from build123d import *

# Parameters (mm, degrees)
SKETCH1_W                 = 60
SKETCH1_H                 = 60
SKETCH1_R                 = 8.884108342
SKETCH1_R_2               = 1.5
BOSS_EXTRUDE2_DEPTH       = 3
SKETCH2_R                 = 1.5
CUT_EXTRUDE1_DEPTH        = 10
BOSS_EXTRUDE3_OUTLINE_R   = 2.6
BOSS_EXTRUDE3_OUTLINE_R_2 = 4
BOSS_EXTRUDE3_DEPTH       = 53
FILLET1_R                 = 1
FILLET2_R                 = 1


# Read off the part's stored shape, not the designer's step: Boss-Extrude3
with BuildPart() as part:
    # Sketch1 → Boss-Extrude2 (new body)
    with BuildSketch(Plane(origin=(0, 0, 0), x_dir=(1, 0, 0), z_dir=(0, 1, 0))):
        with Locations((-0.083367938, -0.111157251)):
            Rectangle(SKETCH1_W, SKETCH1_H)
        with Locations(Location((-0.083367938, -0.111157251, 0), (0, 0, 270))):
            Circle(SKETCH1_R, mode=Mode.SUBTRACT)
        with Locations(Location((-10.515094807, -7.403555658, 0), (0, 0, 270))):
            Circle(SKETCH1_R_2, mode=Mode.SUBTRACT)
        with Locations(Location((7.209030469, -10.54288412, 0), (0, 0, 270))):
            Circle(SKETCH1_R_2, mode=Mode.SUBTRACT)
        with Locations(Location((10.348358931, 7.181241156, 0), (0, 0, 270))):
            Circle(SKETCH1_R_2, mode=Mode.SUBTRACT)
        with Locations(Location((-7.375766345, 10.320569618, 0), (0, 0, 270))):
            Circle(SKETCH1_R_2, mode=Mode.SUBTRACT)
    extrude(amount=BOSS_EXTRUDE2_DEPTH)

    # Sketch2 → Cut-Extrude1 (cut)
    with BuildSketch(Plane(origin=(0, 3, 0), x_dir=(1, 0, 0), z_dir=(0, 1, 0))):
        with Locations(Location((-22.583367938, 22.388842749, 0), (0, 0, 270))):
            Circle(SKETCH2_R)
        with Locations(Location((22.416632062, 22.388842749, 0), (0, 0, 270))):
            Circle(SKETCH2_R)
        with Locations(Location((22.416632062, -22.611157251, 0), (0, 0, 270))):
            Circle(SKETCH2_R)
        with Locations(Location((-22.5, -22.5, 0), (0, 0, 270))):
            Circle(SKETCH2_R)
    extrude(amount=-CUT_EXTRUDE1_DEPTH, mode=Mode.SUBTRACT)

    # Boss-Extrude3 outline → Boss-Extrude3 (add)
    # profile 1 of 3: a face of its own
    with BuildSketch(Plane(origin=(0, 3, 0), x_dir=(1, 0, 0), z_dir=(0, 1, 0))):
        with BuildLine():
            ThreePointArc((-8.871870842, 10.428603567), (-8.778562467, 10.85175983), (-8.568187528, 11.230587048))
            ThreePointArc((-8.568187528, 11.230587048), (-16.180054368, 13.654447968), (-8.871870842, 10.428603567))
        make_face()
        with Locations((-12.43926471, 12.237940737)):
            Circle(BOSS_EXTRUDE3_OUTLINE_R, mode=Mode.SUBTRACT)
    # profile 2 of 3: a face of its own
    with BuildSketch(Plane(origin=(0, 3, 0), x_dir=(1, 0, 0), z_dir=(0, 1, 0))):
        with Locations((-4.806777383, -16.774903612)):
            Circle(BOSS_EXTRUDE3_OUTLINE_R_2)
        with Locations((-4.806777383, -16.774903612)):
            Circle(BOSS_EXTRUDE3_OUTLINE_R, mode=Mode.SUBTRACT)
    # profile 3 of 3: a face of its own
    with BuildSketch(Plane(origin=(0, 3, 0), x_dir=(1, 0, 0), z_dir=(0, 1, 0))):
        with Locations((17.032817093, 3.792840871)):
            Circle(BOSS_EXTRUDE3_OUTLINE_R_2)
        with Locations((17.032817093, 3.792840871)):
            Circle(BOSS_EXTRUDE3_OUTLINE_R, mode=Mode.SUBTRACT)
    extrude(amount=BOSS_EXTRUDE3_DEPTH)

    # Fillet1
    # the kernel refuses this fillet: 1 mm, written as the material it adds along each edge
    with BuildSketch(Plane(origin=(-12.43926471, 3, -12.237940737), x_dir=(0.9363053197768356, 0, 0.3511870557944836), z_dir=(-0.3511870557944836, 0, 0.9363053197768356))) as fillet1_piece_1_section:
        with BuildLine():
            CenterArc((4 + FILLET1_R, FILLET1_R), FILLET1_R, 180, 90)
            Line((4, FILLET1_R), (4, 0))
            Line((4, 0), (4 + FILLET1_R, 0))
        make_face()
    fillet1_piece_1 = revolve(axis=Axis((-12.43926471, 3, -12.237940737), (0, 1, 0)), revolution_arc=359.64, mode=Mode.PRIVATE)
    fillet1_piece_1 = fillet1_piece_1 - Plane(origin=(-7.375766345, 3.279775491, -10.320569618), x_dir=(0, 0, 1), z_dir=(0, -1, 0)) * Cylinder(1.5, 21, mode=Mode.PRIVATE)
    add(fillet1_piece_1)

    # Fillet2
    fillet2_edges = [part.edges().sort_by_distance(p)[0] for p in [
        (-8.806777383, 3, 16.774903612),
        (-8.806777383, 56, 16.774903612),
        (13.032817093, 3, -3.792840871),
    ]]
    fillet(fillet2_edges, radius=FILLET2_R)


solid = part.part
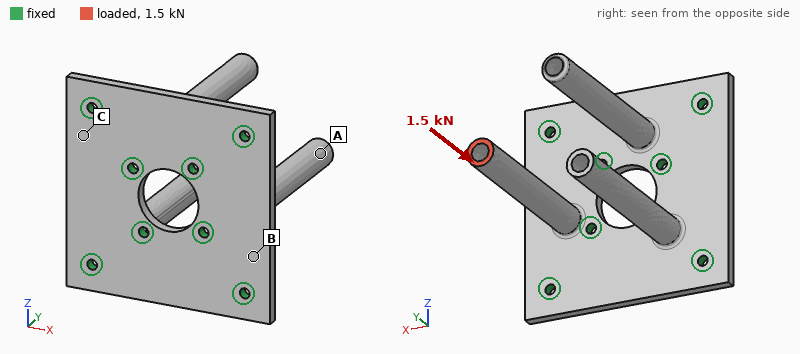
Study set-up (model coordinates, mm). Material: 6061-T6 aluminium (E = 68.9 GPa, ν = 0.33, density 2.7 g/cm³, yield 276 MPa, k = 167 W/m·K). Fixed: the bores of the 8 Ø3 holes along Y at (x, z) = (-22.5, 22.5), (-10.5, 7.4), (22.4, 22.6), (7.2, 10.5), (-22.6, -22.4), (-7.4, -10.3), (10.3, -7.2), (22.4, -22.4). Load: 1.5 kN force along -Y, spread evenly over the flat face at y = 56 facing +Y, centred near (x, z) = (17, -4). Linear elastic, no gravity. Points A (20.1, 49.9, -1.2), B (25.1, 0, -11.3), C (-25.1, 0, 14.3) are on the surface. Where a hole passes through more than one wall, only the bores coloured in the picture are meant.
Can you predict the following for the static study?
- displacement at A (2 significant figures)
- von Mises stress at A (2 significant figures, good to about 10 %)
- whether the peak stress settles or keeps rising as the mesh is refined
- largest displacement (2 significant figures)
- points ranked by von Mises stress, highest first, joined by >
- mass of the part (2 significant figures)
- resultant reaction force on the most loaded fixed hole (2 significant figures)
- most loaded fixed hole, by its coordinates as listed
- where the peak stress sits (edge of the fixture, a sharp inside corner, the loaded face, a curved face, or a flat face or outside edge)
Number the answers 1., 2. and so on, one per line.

1. 0.25 mm
2. 52 MPa
3. keeps rising
4. 0.28 mm
5. A > B > C
6. 39 g
7. 1.1 kN
8. (10.3, -7.2)
9. edge of the fixture
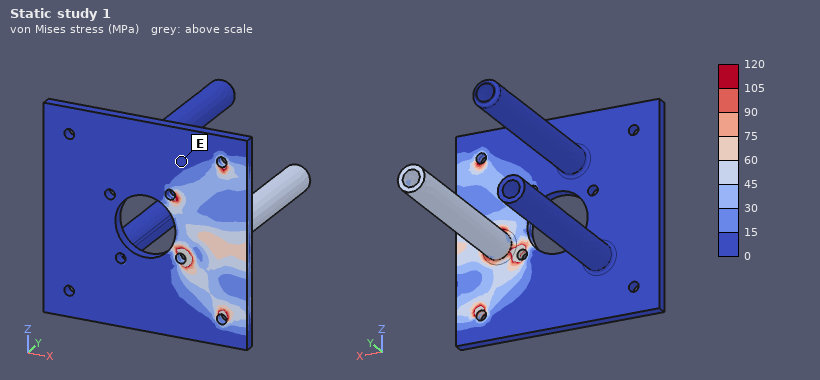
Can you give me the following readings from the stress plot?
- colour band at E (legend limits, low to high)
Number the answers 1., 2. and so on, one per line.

1. 0 to 15 MPa
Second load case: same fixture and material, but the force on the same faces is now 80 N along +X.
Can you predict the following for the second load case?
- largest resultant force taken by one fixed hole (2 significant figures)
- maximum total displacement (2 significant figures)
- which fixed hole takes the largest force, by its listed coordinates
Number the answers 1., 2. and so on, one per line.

1. 170 N
2. 0.55 mm
3. (10.3, -7.2)
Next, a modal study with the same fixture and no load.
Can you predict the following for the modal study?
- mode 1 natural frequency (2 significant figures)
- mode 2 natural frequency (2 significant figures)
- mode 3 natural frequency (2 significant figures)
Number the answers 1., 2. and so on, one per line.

1. 1800 Hz
2. 1800 Hz
3. 2000 Hz
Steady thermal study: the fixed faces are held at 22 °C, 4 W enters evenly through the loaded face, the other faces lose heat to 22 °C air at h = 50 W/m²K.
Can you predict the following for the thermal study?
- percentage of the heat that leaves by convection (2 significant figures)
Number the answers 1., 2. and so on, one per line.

1. 44 %
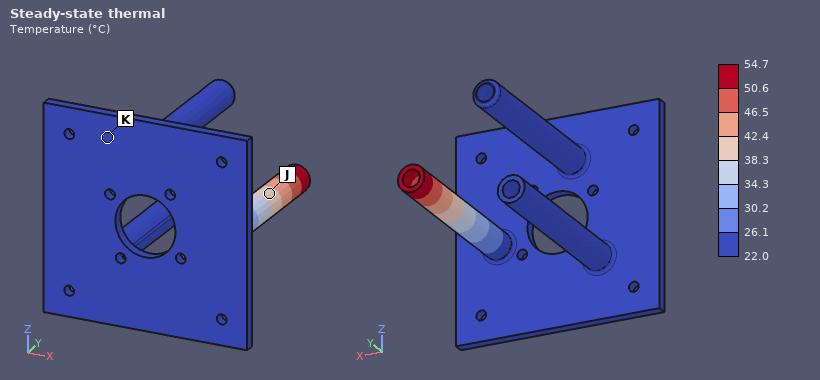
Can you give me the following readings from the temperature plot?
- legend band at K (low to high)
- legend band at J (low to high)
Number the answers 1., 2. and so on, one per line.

1. 22.0 to 26.1 °C
2. 38.3 to 42.4 °C
